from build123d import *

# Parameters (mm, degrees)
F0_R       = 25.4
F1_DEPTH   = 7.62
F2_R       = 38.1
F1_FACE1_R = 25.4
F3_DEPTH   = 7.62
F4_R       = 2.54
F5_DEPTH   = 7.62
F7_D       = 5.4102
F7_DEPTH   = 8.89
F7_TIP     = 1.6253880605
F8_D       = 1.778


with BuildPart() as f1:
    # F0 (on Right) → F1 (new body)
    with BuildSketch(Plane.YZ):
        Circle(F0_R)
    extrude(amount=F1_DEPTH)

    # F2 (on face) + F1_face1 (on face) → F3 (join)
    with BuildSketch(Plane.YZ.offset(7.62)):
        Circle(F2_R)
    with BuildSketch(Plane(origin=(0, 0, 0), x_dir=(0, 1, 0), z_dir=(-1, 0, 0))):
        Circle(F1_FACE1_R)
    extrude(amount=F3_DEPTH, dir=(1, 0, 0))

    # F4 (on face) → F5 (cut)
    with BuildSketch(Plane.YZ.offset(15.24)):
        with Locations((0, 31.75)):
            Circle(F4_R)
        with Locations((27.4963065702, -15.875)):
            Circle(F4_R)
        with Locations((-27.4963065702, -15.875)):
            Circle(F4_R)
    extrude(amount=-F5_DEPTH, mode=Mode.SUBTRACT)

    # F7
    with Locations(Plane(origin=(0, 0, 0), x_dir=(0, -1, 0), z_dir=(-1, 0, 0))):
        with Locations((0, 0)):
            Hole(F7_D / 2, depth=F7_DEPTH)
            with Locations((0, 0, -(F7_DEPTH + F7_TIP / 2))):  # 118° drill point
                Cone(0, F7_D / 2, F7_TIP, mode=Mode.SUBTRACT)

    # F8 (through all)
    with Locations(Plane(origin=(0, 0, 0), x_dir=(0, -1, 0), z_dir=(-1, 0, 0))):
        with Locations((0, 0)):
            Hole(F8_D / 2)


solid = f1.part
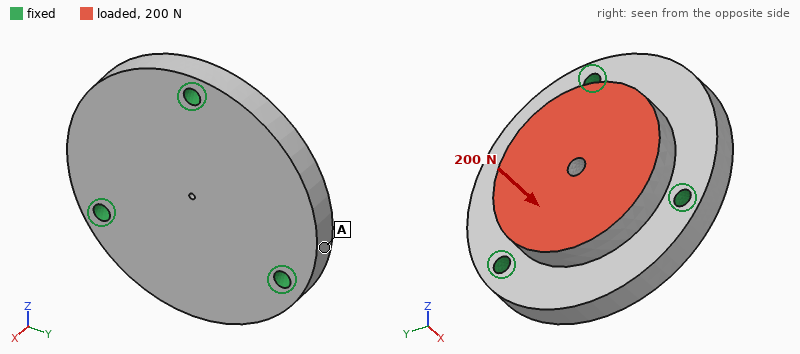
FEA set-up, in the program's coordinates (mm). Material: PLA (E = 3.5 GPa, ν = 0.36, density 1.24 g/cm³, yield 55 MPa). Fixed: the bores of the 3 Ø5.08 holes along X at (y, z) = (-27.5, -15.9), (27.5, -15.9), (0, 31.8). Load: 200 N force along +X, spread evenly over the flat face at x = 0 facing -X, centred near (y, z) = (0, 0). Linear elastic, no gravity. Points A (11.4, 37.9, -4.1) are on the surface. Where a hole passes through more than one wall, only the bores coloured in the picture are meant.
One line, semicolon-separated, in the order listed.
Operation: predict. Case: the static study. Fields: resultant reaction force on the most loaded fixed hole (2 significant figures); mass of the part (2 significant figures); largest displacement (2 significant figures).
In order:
73 N; 61 g; 9.3 µm
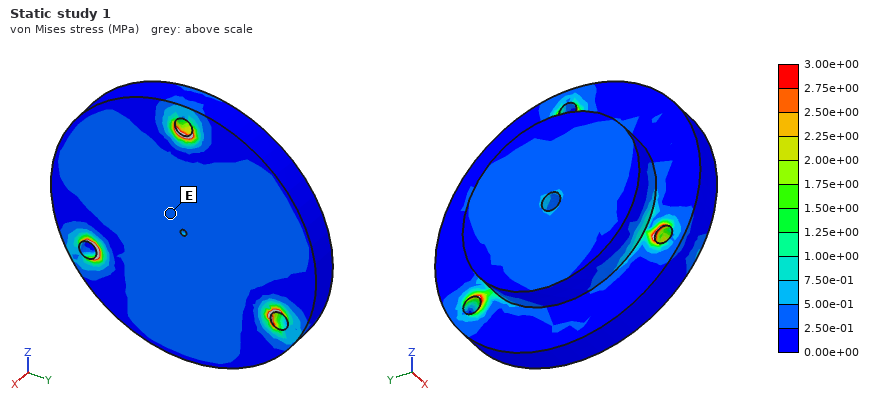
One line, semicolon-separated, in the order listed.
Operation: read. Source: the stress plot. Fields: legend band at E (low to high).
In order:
2.50e-01 to 5.00e-01 MPa
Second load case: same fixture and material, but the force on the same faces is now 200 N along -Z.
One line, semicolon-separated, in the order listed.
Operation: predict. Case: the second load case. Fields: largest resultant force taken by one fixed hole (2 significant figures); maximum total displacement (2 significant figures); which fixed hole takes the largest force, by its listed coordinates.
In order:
96 N; 11 µm; (0, 31.8)
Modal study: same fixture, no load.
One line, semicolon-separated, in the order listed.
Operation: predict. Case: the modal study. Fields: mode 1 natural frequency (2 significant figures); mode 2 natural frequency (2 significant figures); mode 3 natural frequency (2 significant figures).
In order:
3400 Hz; 3400 Hz; 3400 Hz
